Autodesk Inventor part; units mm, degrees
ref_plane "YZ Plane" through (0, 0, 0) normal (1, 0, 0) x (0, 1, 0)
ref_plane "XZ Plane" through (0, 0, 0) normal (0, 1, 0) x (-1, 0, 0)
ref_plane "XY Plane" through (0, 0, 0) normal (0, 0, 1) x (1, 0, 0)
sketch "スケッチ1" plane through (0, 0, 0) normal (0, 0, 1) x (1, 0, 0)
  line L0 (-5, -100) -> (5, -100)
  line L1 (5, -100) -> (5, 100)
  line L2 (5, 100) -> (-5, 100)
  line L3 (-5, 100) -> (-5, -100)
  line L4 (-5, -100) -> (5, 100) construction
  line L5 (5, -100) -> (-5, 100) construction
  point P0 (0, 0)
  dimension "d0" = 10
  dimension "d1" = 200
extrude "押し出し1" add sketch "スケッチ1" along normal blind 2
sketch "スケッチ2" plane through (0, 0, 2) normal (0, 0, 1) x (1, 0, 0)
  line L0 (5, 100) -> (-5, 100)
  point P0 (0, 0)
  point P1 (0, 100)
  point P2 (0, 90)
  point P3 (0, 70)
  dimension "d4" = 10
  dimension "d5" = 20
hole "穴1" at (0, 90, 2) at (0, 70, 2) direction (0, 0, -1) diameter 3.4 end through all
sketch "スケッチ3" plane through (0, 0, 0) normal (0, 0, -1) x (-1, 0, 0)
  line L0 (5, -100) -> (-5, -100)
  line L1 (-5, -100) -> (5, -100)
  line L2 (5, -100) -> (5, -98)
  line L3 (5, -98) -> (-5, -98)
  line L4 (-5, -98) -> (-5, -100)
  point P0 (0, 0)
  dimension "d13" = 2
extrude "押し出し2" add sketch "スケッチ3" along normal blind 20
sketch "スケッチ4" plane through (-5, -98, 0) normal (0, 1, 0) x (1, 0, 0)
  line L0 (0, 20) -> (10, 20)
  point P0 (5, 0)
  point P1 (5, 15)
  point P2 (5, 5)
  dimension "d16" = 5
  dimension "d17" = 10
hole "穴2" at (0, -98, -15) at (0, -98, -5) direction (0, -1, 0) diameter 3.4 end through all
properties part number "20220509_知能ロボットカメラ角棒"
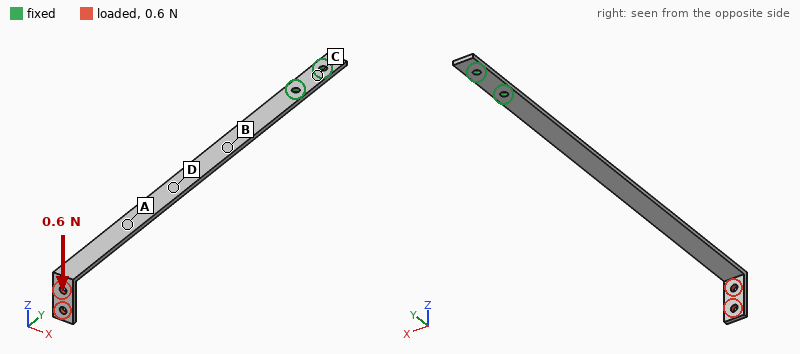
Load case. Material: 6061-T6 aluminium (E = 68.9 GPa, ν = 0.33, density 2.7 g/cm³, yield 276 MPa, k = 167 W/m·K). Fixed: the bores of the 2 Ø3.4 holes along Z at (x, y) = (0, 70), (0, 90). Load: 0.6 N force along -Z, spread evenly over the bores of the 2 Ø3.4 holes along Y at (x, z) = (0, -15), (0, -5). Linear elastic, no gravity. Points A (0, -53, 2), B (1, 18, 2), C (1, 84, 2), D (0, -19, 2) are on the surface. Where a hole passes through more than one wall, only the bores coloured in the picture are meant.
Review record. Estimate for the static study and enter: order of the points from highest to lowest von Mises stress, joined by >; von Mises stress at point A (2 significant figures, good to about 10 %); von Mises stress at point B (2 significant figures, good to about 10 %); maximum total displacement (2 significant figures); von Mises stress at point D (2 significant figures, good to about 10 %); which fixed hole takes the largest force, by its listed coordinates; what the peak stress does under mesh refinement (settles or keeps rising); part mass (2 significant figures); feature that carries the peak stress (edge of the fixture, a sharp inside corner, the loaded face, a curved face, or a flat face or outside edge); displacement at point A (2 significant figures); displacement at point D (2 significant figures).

B > D > A > C
4.1 MPa
11 MPa
2.1 mm
7.2 MPa
(0, 70)
keeps rising
12 g
edge of the fixture
1.2 mm
0.70 mm
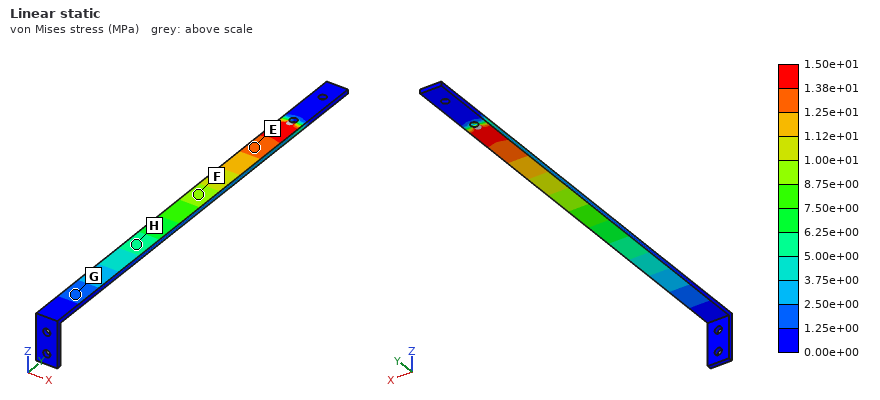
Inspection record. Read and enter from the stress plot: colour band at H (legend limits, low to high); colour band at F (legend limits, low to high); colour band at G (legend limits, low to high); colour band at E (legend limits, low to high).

5.00e+00 to 6.25e+00 MPa
8.75e+00 to 1.00e+01 MPa
1.25e+00 to 2.50e+00 MPa
1.25e+01 to 1.38e+01 MPa
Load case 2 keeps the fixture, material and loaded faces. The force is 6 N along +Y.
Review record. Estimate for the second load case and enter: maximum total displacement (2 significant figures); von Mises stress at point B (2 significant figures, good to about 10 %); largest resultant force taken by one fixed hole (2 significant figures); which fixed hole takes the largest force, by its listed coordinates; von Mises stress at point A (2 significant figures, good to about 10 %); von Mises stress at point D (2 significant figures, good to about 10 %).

2.1 mm
9.6 MPa
5.7 N
(0, 70)
9.6 MPa
9.6 MPa
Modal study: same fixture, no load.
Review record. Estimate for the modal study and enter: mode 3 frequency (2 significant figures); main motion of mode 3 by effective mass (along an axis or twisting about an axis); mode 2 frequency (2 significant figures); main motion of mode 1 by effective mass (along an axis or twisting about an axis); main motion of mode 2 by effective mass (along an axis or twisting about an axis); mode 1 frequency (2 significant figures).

310 Hz
along Z
230 Hz
along Z
along X
48 Hz
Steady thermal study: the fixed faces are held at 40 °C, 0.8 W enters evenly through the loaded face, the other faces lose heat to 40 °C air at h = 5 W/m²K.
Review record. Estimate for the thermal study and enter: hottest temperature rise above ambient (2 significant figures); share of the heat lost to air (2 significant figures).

31 K
41 %
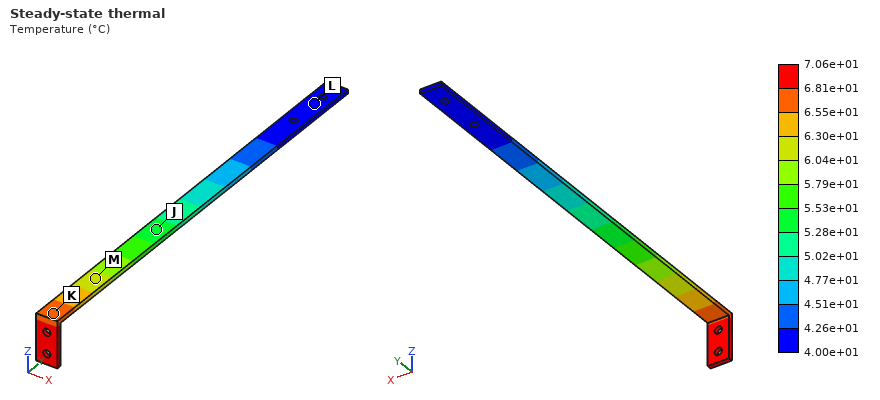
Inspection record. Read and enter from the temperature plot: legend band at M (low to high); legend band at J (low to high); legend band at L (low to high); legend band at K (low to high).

6.04e+01 to 6.30e+01 °C
5.28e+01 to 5.53e+01 °C
4.00e+01 to 4.26e+01 °C
6.55e+01 to 6.81e+01 °C
